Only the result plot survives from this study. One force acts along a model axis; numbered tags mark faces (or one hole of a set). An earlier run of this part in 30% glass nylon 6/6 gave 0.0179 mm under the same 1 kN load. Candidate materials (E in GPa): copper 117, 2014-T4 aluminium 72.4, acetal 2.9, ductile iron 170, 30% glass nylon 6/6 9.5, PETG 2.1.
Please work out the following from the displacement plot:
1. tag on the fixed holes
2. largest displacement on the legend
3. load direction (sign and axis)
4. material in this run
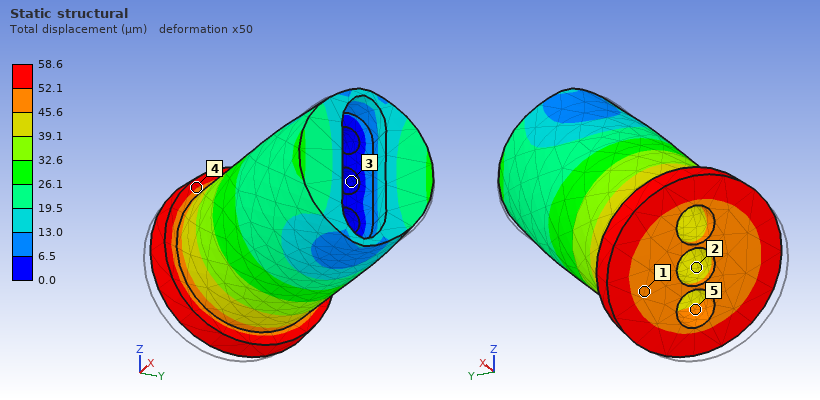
3
58.6 µm
+X
acetal
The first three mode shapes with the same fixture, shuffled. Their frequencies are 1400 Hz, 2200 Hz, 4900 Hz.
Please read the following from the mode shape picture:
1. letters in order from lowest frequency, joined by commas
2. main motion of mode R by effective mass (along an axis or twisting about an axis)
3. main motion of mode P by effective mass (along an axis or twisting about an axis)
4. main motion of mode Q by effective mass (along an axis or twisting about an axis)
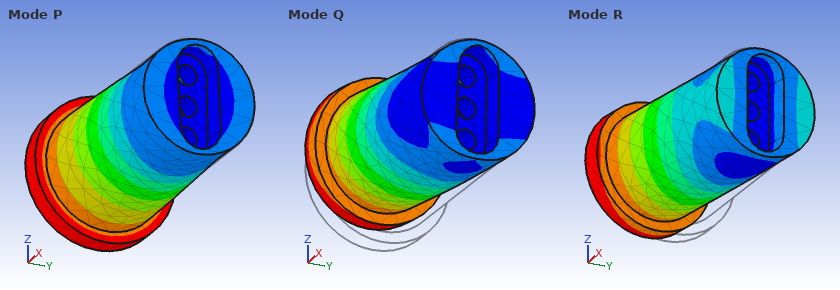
R, Q, P
along Y
twisting about X
along Z
